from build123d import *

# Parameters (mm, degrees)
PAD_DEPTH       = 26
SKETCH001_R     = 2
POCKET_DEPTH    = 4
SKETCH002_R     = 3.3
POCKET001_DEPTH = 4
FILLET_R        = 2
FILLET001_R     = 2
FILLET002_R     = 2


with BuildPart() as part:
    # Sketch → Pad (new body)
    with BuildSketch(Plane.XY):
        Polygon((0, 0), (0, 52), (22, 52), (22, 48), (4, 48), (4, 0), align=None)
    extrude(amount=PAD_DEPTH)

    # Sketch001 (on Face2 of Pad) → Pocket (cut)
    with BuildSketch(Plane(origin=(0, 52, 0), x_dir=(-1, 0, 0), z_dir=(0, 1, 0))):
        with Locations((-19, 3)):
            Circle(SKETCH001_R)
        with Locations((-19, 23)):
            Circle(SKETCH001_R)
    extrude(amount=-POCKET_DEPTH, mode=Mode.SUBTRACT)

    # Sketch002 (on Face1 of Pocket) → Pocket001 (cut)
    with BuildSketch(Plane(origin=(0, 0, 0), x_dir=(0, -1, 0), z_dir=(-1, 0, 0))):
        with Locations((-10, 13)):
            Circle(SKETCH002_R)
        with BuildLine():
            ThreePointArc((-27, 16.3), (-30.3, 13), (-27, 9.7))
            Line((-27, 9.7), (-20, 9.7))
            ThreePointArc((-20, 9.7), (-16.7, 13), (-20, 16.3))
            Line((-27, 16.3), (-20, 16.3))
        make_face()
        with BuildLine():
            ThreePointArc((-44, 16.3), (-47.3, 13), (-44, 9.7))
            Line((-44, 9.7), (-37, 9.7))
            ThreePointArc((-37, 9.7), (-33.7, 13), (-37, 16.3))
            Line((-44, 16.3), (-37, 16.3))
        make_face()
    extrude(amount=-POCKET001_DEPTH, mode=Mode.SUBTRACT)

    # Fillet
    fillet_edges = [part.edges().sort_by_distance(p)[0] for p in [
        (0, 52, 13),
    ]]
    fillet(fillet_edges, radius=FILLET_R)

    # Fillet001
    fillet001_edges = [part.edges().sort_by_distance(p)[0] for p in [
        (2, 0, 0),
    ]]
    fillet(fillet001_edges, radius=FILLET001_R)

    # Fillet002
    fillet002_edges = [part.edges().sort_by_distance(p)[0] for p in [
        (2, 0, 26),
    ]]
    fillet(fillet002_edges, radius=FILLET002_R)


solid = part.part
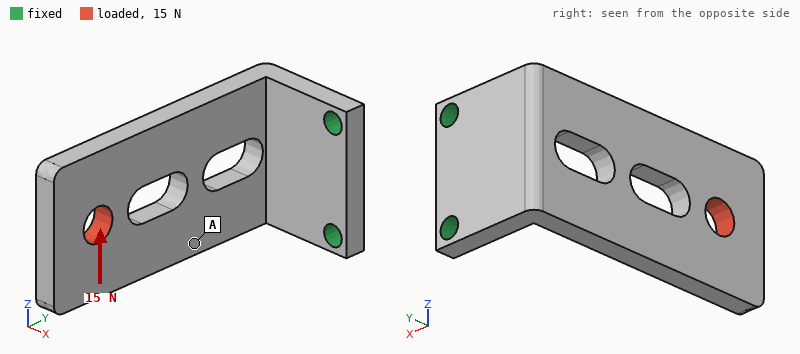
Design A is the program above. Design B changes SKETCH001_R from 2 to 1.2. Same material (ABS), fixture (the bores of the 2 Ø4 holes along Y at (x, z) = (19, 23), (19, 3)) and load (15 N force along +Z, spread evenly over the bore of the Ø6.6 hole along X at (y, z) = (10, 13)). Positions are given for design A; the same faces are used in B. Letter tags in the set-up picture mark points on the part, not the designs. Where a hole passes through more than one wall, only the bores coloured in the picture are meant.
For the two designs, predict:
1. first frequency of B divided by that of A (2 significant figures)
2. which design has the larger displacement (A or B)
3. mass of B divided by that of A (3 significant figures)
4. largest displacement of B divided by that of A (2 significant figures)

0.97
B
1.01
1.1
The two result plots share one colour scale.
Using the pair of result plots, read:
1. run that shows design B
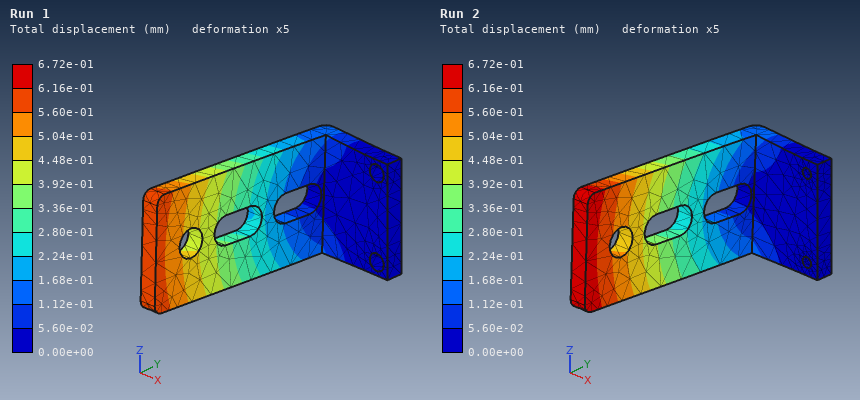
Run 2
